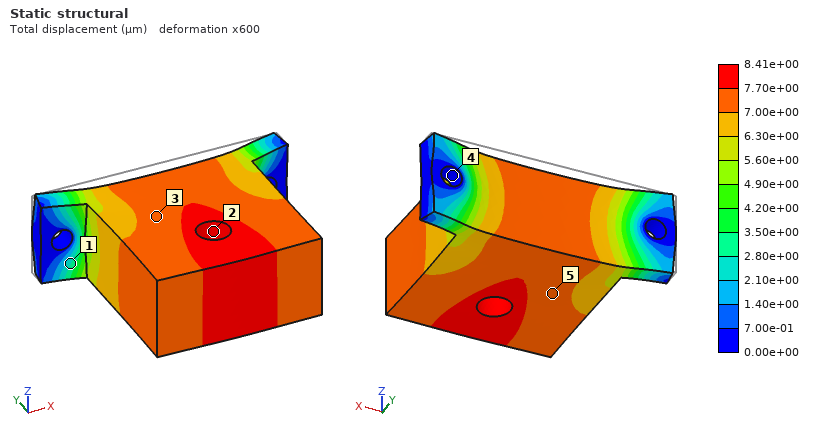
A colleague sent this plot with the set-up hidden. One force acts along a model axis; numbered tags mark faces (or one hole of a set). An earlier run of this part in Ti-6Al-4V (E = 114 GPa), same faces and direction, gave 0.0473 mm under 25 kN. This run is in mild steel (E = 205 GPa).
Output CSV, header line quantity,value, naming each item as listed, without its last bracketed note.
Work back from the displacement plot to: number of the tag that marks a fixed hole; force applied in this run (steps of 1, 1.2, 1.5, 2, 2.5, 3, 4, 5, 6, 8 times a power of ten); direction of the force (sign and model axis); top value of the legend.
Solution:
quantity,value
number of the tag that marks a fixed hole,4
force applied in this run,8 kN
direction of the force,-Y
top value of the legend,8.41e+00 µm
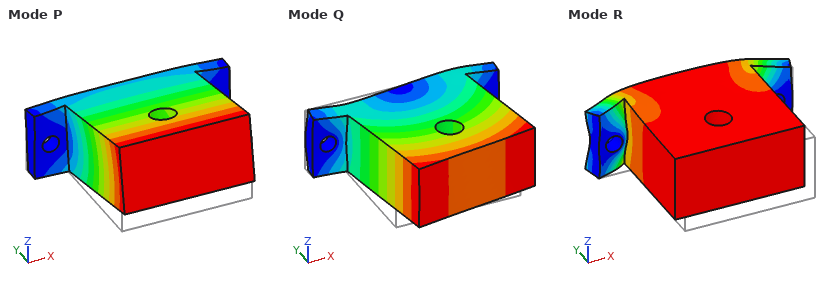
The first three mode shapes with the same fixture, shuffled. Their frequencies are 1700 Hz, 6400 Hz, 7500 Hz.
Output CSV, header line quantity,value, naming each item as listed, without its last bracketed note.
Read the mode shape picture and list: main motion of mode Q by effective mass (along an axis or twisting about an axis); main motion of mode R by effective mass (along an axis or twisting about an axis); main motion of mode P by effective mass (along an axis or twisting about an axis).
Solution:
quantity,value
main motion of mode Q by effective mass,along X
main motion of mode R by effective mass,along Y
main motion of mode P by effective mass,along Z
